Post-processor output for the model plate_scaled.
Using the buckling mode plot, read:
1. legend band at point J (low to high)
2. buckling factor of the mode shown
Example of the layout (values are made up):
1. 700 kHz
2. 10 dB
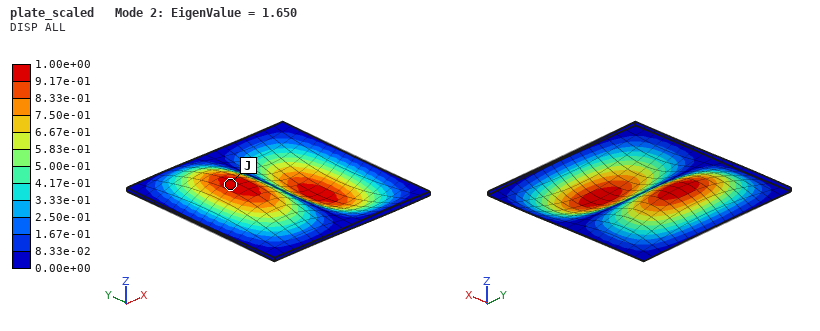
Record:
1. 9.17e-01 to 1.00e+00
2. 1.650
